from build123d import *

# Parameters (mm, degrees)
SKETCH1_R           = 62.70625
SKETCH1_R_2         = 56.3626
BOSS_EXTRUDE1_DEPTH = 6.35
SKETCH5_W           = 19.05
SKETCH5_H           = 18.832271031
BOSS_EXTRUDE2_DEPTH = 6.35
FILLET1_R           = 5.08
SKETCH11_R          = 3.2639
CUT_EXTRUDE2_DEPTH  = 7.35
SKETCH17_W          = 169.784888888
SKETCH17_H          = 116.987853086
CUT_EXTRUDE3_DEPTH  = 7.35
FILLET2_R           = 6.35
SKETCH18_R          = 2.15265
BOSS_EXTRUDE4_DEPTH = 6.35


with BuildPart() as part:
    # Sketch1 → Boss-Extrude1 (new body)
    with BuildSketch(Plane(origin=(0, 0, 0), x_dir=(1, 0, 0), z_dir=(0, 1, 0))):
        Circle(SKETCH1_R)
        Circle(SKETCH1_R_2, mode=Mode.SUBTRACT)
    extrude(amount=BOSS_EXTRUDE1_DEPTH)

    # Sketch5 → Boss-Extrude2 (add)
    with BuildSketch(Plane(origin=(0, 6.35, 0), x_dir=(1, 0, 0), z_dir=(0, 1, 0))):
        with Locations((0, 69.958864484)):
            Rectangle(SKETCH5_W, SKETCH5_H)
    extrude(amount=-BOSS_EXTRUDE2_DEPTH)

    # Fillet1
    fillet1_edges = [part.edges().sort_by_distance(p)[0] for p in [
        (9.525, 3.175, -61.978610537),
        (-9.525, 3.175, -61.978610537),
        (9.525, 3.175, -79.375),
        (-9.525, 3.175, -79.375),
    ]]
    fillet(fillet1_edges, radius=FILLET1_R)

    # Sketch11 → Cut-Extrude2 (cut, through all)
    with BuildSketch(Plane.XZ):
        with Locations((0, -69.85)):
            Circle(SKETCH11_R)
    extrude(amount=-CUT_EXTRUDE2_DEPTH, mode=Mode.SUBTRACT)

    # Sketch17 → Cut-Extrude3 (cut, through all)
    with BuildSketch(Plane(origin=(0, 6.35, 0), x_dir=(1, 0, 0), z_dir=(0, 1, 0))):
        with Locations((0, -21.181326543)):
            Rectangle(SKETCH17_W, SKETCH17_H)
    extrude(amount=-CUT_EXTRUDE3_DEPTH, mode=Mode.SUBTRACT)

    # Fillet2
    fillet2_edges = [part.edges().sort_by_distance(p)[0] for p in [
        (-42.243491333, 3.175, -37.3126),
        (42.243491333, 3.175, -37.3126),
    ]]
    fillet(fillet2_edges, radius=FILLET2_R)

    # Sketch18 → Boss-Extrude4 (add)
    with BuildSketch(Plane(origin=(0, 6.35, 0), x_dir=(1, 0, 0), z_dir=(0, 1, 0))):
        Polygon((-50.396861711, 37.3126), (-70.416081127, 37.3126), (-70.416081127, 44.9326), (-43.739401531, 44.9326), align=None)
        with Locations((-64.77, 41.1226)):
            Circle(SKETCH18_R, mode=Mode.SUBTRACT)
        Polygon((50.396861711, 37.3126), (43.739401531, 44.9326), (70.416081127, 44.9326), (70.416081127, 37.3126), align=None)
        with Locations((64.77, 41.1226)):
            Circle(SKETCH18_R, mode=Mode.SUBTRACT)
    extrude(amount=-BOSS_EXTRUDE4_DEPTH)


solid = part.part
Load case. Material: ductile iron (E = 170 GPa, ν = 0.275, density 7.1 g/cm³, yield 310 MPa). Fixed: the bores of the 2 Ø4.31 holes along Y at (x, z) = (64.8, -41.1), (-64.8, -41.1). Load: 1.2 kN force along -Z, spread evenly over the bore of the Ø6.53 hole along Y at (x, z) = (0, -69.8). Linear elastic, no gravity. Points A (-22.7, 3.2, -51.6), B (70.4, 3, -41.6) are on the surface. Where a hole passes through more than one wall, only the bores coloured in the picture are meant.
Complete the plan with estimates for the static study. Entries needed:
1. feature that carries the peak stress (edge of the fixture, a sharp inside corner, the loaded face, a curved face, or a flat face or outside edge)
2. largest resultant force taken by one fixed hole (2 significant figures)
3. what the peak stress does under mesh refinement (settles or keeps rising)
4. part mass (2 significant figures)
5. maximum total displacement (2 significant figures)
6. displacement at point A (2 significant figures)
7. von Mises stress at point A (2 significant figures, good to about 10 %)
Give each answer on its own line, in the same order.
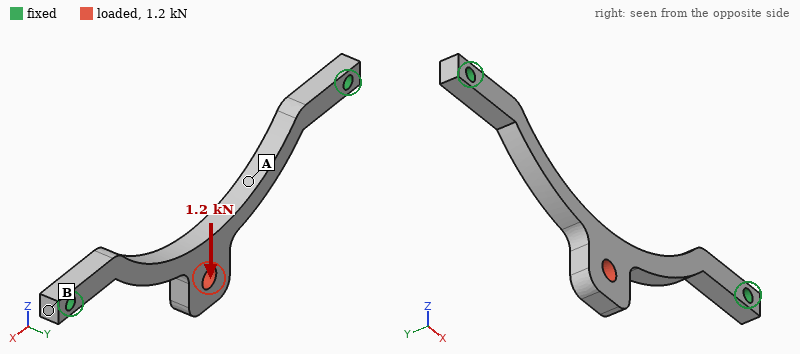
edge of the fixture
1.4 kN
keeps rising
58 g
53 µm
43 µm
51 MPa
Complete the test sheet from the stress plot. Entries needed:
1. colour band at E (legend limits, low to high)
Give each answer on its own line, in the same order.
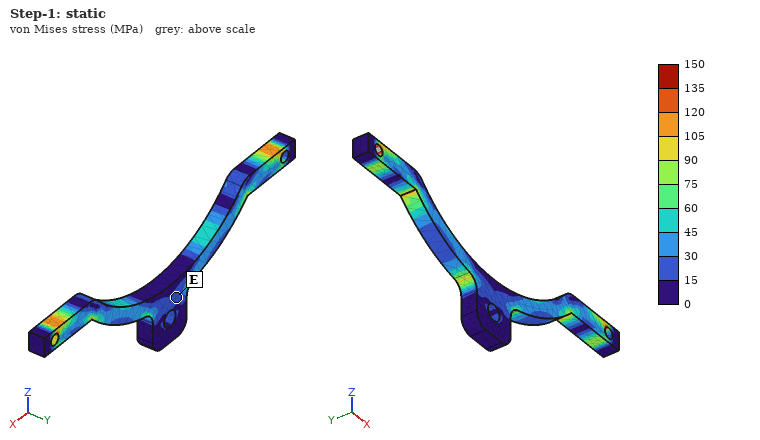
15 to 30 MPa
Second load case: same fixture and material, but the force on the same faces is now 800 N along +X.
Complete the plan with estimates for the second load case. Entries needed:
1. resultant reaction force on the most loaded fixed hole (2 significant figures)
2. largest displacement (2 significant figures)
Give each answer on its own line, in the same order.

460 N
27 µm
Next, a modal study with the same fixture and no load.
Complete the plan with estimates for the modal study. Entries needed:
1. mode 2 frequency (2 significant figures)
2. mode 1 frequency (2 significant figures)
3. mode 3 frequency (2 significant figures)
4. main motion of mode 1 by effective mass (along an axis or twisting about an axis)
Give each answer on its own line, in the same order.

4000 Hz
1000 Hz
4100 Hz
along Y
